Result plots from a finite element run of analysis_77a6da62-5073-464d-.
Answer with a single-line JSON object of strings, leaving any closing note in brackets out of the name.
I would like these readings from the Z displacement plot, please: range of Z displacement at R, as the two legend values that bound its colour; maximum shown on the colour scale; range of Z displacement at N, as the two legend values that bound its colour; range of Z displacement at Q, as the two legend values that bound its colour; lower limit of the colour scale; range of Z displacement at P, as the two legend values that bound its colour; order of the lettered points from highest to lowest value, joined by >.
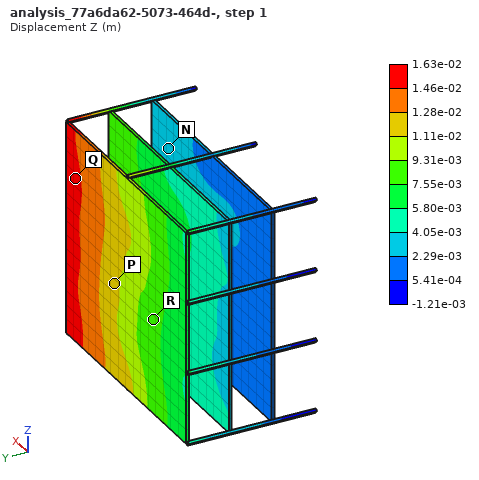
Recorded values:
{"range of Z displacement at R, as the two legend values that bound its colour": "7.55e-03 to 9.31e-03 m", "maximum shown on the colour scale": "1.63e-02 m", "range of Z displacement at N, as the two legend values that bound its colour": "2.29e-03 to 4.05e-03 m", "range of Z displacement at Q, as the two legend values that bound its colour": "1.46e-02 to 1.63e-02 m", "lower limit of the colour scale": "-1.21e-03 m", "range of Z displacement at P, as the two legend values that bound its colour": "1.11e-02 to 1.28e-02 m", "order of the lettered points from highest to lowest value, joined by >": "Q > P > R > N"}
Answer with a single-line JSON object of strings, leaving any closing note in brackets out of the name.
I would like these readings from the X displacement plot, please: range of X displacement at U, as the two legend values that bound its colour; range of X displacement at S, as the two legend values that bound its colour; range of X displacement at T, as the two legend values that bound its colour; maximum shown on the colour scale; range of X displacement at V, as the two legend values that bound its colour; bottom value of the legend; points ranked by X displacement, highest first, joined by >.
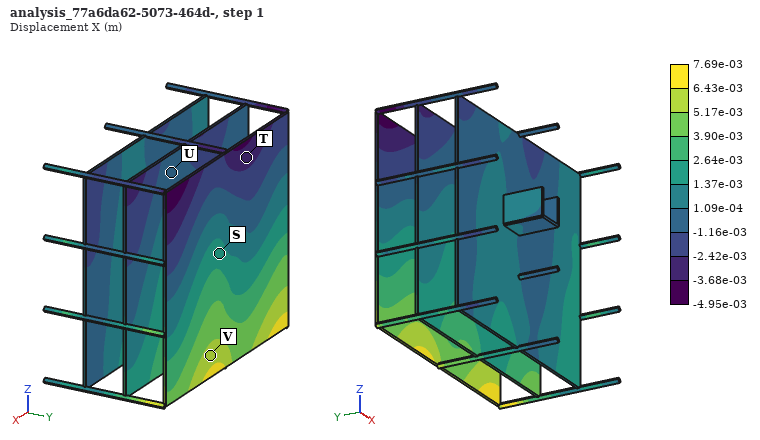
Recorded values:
{"range of X displacement at U, as the two legend values that bound its colour": "-1.16e-03 to 1.09e-04 m", "range of X displacement at S, as the two legend values that bound its colour": "1.37e-03 to 2.64e-03 m", "range of X displacement at T, as the two legend values that bound its colour": "-3.68e-03 to -2.42e-03 m", "maximum shown on the colour scale": "7.69e-03 m", "range of X displacement at V, as the two legend values that bound its colour": "5.17e-03 to 6.43e-03 m", "bottom value of the legend": "-4.95e-03 m", "points ranked by X displacement, highest first, joined by >": "V > S > U > T"}
